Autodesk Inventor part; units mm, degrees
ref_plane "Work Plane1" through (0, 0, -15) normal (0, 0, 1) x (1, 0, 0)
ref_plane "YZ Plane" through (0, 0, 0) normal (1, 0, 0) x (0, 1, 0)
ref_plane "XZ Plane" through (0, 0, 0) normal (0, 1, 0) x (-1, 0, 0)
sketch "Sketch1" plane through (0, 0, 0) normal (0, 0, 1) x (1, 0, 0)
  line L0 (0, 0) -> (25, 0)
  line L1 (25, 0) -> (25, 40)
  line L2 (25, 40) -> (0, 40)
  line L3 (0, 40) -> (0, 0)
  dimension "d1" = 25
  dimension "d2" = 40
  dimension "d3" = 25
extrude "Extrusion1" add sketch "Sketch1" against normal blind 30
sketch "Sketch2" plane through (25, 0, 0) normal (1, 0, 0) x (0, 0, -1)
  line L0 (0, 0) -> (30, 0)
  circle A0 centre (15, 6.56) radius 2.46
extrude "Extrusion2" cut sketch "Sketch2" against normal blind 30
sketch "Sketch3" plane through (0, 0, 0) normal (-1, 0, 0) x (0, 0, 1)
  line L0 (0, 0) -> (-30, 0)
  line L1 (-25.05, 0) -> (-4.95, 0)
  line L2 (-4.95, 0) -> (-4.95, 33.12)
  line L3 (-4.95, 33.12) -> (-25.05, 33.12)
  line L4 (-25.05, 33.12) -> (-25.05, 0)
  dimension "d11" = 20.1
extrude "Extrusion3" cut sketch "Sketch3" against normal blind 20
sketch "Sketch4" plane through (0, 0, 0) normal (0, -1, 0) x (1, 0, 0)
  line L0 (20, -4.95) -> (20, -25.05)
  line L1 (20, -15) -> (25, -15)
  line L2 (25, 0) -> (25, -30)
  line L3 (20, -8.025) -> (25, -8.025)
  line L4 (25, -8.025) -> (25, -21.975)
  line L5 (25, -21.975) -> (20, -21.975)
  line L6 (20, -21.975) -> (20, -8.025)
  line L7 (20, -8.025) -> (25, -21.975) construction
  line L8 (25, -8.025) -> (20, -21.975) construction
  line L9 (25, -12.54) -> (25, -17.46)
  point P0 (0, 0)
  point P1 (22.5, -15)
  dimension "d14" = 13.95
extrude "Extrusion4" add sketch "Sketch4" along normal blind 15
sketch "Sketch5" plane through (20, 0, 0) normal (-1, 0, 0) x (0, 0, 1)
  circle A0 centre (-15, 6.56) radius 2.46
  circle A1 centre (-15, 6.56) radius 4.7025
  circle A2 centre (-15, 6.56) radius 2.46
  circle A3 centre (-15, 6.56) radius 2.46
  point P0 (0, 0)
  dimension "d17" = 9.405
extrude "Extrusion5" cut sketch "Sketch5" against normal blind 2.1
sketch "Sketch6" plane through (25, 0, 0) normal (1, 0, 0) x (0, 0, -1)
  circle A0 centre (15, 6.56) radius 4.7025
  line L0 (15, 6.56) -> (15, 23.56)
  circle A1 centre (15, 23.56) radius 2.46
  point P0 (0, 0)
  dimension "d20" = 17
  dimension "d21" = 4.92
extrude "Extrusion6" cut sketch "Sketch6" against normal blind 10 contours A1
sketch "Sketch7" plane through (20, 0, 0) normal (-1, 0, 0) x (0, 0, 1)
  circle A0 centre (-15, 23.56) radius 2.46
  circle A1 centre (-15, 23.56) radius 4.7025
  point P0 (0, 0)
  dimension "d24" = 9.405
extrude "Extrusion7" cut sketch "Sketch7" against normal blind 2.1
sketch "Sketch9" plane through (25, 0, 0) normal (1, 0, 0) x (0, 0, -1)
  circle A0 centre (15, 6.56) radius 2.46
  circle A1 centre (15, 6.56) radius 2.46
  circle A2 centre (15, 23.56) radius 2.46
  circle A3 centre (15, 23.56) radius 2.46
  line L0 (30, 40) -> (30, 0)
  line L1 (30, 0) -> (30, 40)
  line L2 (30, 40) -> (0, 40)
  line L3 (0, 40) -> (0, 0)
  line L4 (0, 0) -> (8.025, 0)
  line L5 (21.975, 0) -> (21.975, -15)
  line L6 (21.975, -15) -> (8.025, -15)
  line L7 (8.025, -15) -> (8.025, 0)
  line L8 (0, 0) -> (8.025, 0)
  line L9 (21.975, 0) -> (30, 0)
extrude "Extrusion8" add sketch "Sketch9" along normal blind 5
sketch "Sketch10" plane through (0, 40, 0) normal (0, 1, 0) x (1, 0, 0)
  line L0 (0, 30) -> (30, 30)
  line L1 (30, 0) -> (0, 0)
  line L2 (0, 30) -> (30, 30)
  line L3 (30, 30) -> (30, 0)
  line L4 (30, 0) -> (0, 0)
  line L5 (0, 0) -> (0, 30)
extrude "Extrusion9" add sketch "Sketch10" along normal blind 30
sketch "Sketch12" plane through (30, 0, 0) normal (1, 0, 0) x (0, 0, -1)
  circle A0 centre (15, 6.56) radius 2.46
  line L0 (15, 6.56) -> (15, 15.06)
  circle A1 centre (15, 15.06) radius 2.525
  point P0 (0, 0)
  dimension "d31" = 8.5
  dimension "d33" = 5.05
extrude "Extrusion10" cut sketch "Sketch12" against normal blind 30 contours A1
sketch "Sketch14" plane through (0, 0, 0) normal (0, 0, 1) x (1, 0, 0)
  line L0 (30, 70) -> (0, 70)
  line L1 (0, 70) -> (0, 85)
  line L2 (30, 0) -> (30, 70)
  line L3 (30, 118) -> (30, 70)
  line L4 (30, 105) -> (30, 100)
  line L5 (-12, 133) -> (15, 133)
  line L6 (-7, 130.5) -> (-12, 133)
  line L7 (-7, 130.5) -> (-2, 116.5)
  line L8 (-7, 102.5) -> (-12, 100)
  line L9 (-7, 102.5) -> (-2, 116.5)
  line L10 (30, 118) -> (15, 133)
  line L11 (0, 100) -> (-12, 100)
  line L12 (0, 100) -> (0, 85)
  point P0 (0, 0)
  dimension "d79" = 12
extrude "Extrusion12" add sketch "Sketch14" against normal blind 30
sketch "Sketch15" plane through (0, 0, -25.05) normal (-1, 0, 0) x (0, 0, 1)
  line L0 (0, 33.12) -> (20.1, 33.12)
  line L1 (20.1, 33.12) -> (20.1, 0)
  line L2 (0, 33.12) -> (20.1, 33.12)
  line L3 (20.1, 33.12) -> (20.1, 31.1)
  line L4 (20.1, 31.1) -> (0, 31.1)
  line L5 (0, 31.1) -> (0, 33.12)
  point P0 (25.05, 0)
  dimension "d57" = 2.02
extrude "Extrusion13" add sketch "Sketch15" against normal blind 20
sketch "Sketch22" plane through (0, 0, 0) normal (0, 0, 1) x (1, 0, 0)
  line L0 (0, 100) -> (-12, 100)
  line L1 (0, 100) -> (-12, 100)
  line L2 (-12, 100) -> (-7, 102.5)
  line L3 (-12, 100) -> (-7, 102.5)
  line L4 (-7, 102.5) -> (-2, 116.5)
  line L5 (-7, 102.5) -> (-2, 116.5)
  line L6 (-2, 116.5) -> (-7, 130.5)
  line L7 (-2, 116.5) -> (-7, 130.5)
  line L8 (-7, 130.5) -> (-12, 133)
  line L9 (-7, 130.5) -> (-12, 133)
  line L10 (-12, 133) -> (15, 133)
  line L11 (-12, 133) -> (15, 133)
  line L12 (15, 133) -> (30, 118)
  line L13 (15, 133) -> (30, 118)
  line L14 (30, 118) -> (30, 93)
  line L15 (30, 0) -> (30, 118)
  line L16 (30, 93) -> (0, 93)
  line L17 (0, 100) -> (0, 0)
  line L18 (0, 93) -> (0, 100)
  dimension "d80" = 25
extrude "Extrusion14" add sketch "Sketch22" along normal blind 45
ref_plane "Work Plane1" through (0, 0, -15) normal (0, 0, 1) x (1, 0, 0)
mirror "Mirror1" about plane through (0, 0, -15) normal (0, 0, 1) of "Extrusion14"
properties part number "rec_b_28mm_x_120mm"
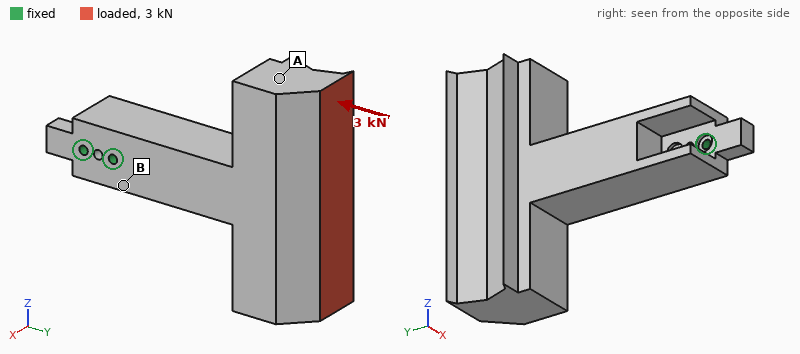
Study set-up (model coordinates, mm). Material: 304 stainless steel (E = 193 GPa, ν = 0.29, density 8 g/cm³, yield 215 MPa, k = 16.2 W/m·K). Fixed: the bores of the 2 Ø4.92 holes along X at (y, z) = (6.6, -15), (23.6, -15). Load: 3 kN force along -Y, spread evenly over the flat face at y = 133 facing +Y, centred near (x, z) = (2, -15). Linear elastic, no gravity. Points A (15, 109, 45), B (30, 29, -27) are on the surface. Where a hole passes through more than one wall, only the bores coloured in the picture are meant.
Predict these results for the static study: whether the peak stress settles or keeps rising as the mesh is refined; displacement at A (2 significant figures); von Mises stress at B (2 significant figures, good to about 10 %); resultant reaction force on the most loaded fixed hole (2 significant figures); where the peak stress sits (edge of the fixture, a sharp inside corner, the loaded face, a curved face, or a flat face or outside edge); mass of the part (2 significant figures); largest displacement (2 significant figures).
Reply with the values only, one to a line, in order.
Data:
keeps rising
58 µm
18 MPa
3.4 kN
edge of the fixture
1.8 kg
83 µm
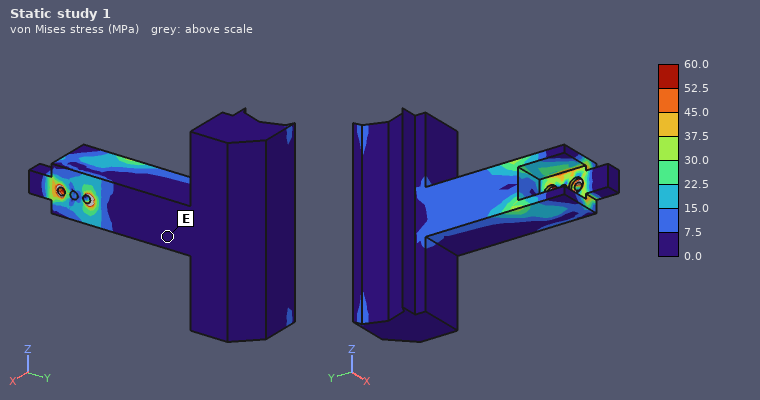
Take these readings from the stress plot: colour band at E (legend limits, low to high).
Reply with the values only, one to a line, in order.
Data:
0.0 to 7.5 MPa
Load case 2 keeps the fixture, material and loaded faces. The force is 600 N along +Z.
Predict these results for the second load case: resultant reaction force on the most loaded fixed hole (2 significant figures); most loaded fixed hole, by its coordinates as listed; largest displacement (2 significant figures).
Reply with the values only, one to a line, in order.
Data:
3.4 kN
(23.6, -15)
70 µm
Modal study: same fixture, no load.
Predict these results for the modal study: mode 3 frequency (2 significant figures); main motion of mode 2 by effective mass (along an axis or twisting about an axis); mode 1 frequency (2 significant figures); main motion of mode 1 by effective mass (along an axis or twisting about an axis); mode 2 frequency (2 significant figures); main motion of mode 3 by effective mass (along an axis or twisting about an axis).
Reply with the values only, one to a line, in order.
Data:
790 Hz
along Z
490 Hz
along X
530 Hz
twisting about Y
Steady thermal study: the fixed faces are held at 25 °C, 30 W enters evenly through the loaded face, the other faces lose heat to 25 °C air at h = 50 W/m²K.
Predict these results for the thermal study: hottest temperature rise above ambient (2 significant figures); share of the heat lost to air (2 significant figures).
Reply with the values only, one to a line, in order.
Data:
46 K
95 %
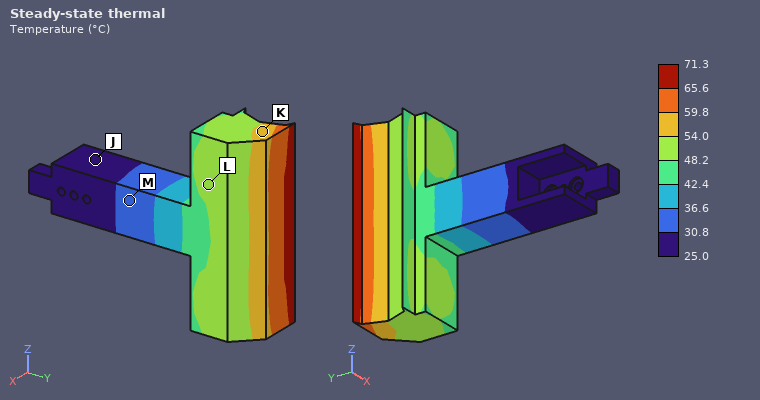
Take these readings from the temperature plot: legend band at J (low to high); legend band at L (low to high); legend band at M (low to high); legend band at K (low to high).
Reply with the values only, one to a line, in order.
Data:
25.0 to 30.8 °C
48.2 to 54.0 °C
30.8 to 36.6 °C
54.0 to 59.8 °C
